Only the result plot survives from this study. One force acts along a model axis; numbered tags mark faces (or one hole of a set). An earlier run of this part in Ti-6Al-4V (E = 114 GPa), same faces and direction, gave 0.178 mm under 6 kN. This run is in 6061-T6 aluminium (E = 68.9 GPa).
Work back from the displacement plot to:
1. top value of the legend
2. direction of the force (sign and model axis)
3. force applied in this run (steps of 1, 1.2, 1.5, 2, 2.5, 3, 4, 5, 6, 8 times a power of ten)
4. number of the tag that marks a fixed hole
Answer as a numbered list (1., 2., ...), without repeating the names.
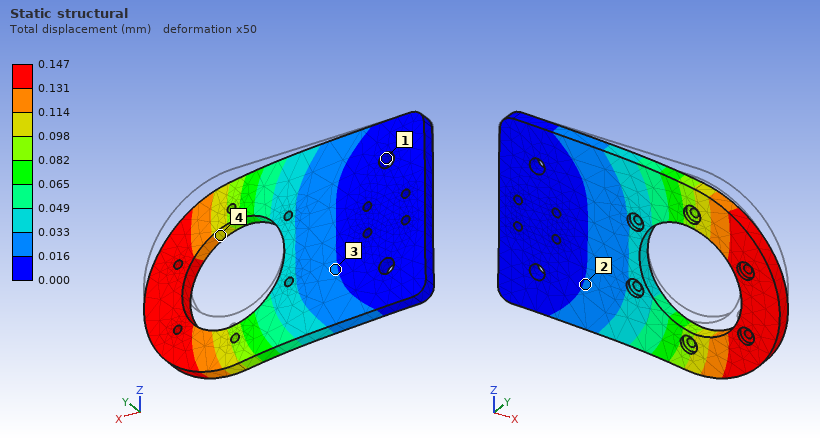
1. 0.147 mm
2. -Z
3. 3 kN
4. 1
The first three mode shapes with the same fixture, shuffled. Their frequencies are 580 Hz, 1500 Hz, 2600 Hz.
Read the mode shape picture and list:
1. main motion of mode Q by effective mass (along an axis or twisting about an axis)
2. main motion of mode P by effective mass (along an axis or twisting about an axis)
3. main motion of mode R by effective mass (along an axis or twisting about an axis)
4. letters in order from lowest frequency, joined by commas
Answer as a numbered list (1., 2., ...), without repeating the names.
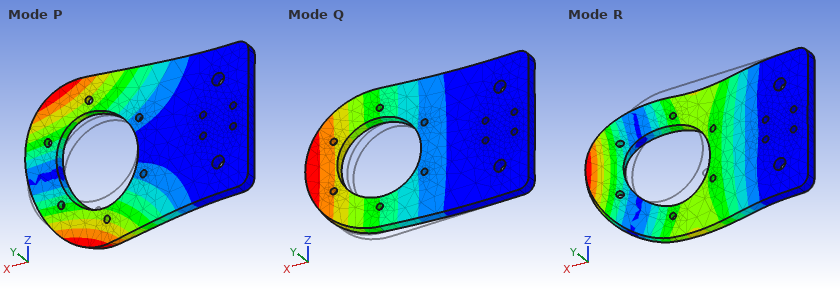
1. along Y
2. twisting about X
3. along Y
4. Q, P, R
